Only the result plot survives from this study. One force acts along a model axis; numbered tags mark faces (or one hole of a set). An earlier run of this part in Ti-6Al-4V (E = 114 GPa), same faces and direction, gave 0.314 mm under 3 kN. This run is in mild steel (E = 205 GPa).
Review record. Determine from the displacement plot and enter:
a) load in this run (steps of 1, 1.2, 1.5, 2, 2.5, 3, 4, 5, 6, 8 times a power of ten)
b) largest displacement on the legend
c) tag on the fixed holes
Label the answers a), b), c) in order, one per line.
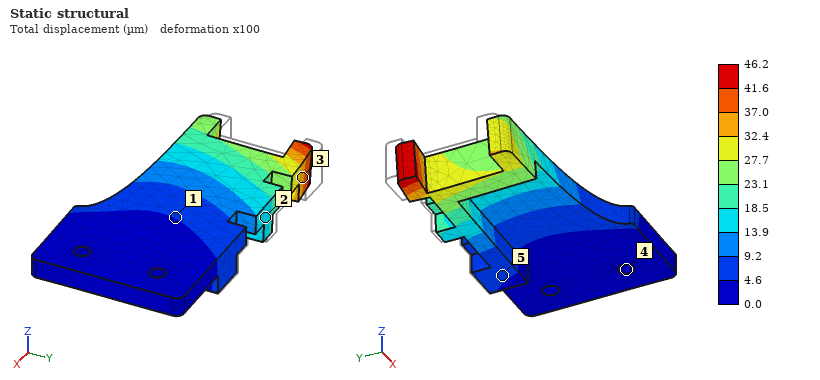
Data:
a) 800 N
b) 46.2 µm
c) 4
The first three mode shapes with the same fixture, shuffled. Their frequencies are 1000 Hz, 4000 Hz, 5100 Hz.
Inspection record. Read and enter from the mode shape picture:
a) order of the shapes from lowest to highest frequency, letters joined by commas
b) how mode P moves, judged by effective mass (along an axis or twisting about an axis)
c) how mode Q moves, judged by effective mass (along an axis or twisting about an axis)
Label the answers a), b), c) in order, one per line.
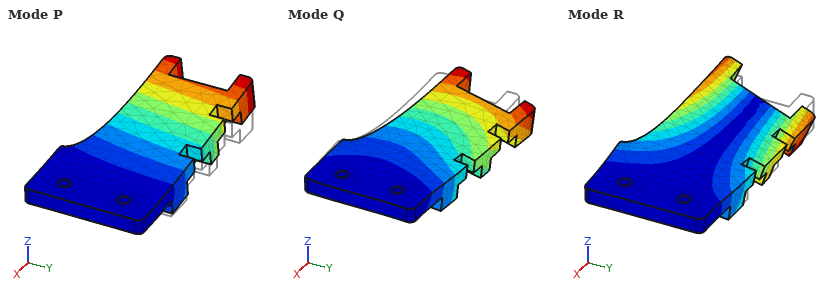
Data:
a) P, R, Q
b) along Z
c) along Y
